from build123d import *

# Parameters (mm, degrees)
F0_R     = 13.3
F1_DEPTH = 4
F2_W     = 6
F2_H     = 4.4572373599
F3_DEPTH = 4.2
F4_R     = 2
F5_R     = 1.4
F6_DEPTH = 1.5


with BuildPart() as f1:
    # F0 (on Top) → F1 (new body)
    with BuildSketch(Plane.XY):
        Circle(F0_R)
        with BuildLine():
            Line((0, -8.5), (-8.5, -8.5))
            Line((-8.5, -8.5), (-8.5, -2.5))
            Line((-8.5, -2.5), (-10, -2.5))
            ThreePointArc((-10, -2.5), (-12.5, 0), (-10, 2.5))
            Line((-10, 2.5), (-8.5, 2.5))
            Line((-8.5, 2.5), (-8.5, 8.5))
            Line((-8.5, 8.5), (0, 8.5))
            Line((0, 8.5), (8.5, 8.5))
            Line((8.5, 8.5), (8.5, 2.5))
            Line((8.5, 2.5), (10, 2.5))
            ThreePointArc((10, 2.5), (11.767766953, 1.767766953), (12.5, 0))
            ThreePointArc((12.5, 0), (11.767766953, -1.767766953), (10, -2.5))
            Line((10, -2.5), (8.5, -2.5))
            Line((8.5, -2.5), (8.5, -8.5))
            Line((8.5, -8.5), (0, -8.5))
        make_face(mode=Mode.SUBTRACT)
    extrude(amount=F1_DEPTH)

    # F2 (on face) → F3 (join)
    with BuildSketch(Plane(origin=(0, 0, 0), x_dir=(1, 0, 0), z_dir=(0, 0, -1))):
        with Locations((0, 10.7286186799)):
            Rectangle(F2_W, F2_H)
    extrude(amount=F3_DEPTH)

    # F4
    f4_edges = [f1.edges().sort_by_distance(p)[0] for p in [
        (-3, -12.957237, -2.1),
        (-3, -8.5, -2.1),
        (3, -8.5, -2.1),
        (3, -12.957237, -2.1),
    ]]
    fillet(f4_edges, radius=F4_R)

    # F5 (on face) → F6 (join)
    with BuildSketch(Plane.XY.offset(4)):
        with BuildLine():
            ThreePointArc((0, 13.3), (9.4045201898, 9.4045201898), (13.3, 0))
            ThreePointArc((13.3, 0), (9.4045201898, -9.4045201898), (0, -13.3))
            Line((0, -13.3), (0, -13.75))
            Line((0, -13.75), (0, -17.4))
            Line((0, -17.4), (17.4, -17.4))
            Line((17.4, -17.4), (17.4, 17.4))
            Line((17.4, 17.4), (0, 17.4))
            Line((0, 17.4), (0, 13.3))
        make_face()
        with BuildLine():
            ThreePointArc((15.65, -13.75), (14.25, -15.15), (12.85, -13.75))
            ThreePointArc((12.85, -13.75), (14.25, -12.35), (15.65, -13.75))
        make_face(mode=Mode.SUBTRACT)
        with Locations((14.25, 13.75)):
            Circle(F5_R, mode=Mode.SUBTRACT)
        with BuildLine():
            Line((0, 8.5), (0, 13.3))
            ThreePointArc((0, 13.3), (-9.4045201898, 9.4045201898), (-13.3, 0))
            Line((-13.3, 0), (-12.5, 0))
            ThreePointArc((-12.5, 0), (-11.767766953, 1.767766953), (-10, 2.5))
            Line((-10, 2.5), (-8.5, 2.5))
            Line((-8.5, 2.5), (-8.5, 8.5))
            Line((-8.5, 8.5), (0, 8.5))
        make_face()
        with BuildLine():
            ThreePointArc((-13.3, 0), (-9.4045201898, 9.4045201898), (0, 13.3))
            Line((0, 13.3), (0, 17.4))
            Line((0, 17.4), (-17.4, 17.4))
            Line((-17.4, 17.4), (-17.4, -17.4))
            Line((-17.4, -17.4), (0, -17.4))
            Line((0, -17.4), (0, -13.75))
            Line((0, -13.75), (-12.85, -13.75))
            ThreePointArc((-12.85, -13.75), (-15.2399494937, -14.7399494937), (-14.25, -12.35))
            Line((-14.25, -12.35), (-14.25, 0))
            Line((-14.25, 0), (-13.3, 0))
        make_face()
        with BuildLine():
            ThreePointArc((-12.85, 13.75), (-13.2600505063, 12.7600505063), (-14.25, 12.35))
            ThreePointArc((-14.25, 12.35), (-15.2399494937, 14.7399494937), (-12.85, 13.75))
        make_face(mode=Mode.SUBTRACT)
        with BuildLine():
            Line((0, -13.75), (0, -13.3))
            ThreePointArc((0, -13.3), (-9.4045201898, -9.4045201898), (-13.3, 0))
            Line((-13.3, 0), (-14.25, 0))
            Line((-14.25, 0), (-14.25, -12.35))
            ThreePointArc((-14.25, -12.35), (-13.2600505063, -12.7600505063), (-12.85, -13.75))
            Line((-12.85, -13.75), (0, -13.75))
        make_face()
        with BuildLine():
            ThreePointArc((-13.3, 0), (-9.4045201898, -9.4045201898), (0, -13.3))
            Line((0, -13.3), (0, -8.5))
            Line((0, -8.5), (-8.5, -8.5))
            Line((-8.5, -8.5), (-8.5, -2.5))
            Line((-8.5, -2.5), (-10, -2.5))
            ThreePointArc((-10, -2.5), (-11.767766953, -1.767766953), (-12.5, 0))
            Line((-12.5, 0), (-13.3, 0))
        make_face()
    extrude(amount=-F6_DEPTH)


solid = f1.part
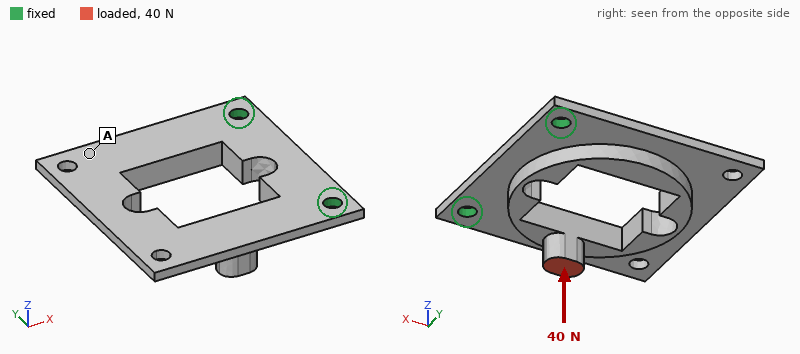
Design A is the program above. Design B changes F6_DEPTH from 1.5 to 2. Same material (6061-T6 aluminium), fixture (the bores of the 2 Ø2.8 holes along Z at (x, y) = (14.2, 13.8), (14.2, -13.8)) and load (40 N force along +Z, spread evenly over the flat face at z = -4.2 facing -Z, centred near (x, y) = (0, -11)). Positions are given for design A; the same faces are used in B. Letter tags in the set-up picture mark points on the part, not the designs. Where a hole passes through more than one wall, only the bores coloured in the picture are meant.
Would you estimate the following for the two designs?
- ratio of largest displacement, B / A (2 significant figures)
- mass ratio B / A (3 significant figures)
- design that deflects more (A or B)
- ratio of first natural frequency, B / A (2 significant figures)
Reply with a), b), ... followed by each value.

a) 0.54
b) 1.16
c) A
d) 1.3
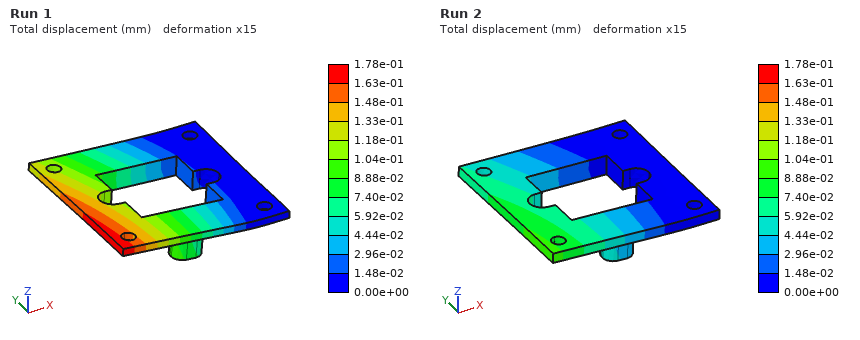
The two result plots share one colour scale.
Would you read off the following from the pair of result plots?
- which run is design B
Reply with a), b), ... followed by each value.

a) Run 2
